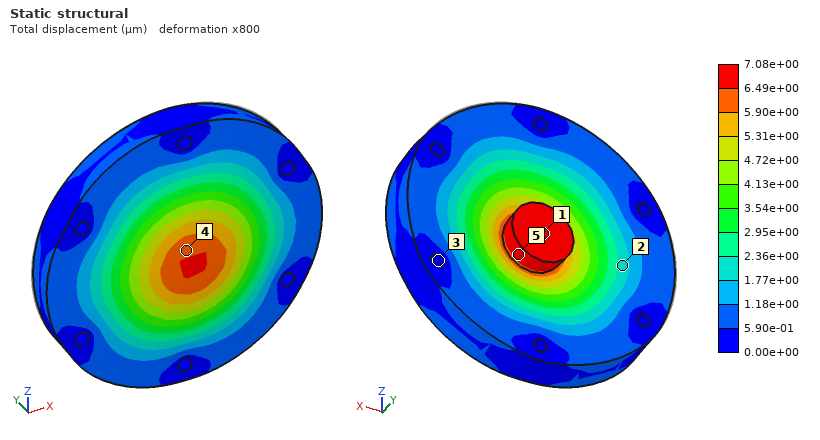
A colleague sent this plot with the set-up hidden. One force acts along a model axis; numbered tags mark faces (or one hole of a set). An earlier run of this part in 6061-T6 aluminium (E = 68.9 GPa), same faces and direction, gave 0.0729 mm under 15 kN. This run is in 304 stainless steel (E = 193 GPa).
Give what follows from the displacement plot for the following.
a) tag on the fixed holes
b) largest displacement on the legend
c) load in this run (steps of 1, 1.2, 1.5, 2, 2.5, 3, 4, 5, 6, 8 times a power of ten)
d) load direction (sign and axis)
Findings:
3
7.08e+00 µm
4 kN
-Y
